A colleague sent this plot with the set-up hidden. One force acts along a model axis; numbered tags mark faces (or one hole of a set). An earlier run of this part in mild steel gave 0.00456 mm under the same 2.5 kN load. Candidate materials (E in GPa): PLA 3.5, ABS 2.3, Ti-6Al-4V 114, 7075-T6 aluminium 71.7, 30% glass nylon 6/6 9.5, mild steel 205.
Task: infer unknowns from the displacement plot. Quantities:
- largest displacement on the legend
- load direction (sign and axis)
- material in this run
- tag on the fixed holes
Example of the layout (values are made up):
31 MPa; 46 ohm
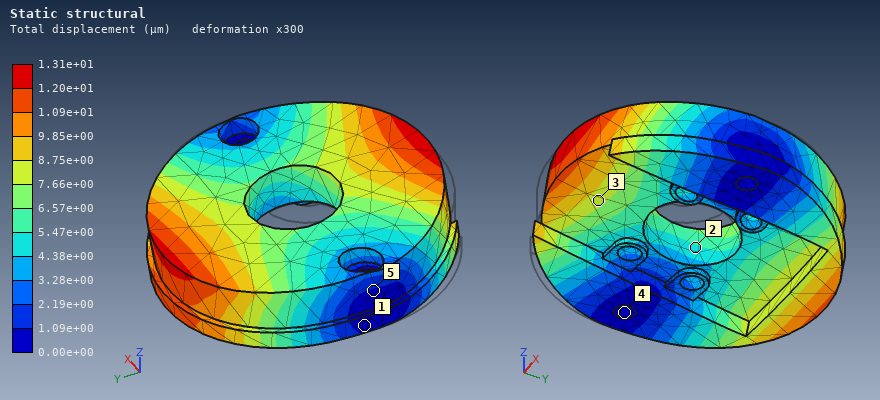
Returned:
1.31e+01 µm; +Y; 7075-T6 aluminium; 4
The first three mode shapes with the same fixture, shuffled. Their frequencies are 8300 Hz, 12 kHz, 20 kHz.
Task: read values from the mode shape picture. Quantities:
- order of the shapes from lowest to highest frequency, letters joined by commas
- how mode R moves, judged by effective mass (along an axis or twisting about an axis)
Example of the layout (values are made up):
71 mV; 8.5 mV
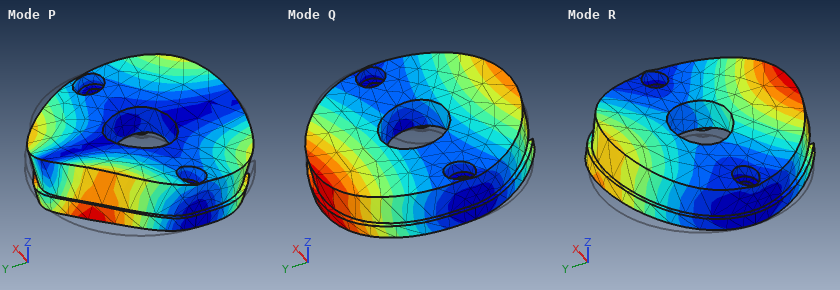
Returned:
Q, R, P; along Z
